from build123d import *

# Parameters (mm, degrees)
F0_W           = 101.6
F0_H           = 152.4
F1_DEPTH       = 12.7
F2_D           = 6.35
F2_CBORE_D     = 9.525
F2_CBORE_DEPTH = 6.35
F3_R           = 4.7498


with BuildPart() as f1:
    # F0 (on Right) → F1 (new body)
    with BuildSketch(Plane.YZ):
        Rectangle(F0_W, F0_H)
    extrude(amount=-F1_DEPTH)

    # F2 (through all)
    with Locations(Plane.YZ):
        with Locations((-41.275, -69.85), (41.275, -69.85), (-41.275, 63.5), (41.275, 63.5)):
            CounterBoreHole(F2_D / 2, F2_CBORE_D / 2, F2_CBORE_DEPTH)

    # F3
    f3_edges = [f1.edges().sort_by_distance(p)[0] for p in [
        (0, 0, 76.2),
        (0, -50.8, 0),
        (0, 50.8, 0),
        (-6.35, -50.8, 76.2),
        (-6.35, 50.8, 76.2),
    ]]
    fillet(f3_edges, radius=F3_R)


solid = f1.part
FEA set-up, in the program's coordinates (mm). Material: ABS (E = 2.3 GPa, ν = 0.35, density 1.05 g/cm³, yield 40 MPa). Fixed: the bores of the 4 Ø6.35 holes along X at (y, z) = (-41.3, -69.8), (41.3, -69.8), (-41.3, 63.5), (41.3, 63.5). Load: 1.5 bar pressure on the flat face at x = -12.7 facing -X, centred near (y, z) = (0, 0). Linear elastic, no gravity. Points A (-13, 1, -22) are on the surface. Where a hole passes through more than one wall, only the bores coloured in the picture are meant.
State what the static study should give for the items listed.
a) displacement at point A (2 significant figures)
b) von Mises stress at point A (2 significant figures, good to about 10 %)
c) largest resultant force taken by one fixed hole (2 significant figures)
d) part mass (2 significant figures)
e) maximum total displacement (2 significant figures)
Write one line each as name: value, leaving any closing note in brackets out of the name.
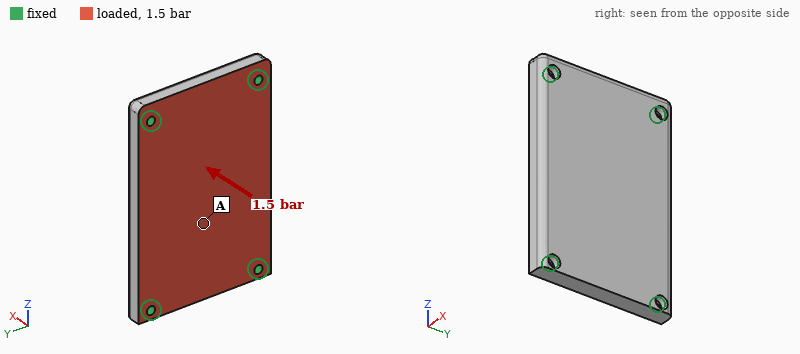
displacement at point A: 0.70 mm
von Mises stress at point A: 4.4 MPa
largest resultant force taken by one fixed hole: 820 N
part mass: 200 g
maximum total displacement: 0.77 mm
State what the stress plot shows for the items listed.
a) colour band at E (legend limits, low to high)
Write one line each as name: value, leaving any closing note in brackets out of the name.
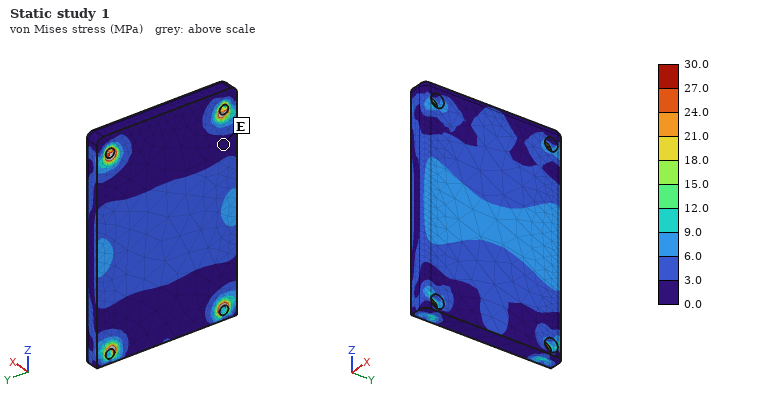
colour band at E: 0.0 to 3.0 MPa
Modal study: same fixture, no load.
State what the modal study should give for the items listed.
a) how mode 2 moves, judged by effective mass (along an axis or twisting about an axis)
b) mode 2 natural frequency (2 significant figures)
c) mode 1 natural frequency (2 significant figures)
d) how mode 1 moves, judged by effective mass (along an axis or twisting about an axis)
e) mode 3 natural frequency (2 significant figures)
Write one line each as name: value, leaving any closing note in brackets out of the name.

how mode 2 moves, judged by effective mass: twisting about Z
mode 2 natural frequency: 1100 Hz
mode 1 natural frequency: 690 Hz
how mode 1 moves, judged by effective mass: along X
mode 3 natural frequency: 1700 Hz
